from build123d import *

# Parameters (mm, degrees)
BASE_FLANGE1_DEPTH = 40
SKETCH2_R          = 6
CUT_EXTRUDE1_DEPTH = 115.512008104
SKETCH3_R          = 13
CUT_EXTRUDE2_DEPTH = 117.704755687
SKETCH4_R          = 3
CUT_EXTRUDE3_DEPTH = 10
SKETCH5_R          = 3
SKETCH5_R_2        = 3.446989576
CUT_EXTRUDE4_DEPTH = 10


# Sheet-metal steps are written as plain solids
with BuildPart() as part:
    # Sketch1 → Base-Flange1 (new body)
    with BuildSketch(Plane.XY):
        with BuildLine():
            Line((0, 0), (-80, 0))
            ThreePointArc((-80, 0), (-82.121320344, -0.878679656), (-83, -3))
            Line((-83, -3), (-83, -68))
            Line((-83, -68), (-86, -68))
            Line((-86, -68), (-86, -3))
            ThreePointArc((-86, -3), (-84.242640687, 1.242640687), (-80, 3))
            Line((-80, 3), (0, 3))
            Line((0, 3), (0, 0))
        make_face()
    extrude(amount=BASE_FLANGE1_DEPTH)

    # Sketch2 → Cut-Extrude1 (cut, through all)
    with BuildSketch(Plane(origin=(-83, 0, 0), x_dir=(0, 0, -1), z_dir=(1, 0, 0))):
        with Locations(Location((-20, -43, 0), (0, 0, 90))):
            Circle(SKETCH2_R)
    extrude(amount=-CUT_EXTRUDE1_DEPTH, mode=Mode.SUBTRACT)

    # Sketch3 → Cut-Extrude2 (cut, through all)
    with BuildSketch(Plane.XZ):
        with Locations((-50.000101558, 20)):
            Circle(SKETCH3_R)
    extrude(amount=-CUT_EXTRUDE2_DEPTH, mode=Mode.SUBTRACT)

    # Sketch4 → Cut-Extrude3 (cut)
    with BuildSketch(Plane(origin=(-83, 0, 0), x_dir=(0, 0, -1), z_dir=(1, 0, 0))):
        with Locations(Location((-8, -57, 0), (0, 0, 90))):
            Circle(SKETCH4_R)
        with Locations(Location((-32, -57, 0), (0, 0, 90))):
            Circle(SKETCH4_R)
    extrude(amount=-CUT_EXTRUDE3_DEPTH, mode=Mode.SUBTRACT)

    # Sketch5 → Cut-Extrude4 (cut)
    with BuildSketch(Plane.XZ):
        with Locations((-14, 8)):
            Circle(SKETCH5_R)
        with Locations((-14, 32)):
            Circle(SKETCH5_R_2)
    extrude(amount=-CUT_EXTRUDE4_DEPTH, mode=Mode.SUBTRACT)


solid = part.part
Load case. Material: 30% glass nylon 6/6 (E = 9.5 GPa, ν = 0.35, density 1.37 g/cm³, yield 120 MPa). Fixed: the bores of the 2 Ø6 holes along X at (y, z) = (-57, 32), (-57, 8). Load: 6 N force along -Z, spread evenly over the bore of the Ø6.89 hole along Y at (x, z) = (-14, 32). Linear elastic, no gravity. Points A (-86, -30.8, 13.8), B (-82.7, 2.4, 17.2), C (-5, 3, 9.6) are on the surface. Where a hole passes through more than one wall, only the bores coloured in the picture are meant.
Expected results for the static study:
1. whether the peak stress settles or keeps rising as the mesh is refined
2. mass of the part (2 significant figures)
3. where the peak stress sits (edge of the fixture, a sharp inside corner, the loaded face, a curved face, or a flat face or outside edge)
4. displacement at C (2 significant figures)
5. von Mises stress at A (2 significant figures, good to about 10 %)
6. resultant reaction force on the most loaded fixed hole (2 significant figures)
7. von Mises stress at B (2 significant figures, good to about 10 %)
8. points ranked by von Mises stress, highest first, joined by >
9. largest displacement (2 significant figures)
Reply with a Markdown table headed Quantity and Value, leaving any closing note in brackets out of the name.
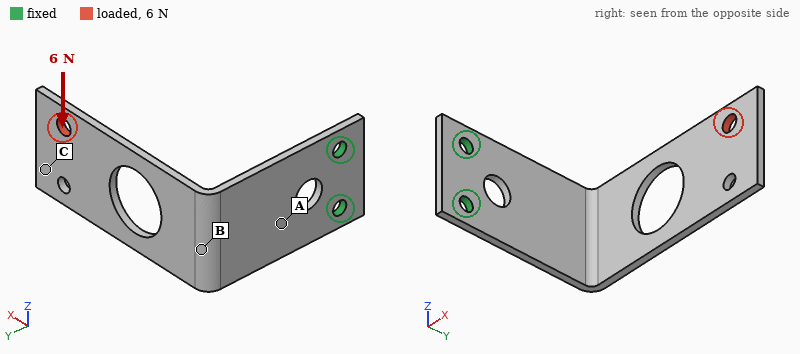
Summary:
| Quantity | Value |
|---|---|
| whether the peak stress settles or keeps rising as the mesh is refined | keeps rising |
| mass of the part | 22 g |
| where the peak stress sits | edge of the fixture |
| displacement at C | 1.3 mm |
| von Mises stress at A | 6.0 MPa |
| resultant reaction force on the most loaded fixed hole | 19 N |
| von Mises stress at B | 2.8 MPa |
| points ranked by von Mises stress, highest first, joined by > | A > B > C |
| largest displacement | 1.4 mm |
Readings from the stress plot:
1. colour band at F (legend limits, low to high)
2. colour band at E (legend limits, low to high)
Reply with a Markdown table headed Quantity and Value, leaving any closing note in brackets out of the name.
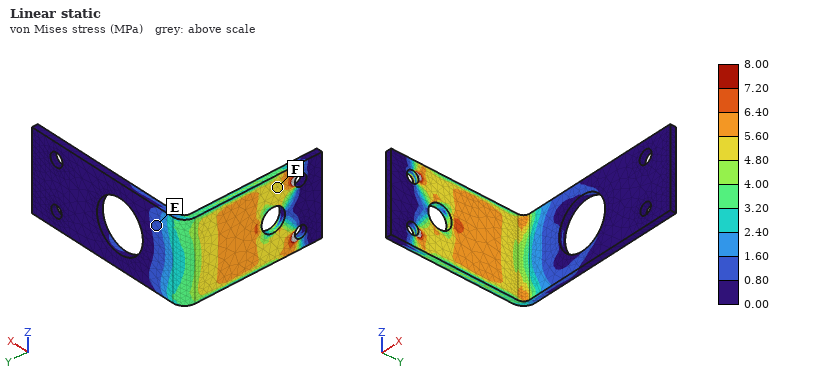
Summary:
| Quantity | Value |
|---|---|
| colour band at F | 4.80 to 5.60 MPa |
| colour band at E | 0.80 to 1.60 MPa |
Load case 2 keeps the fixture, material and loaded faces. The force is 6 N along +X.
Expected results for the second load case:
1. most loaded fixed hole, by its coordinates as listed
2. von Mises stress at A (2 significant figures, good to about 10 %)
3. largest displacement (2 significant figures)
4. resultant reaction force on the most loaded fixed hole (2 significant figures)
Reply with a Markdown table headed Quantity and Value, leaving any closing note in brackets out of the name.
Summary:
| Quantity | Value |
|---|---|
| most loaded fixed hole, by its coordinates as listed | (-57, 32) |
| von Mises stress at A | 3.1 MPa |
| largest displacement | 1.2 mm |
| resultant reaction force on the most loaded fixed hole | 5.3 N |
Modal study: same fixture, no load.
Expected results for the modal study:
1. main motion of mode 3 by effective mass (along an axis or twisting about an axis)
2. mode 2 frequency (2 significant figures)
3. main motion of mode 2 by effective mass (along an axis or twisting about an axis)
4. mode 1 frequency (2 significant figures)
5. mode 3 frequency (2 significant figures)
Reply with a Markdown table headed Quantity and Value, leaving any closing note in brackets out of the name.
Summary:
| Quantity | Value |
|---|---|
| main motion of mode 3 by effective mass | along X |
| mode 2 frequency | 150 Hz |
| main motion of mode 2 by effective mass | along Z |
| mode 1 frequency | 84 Hz |
| mode 3 frequency | 240 Hz |
